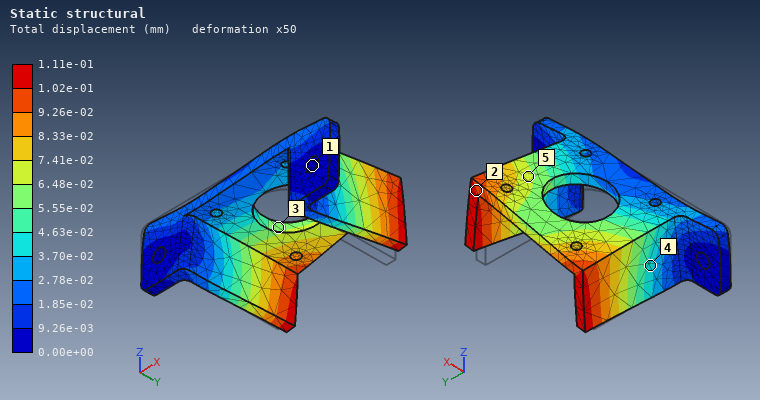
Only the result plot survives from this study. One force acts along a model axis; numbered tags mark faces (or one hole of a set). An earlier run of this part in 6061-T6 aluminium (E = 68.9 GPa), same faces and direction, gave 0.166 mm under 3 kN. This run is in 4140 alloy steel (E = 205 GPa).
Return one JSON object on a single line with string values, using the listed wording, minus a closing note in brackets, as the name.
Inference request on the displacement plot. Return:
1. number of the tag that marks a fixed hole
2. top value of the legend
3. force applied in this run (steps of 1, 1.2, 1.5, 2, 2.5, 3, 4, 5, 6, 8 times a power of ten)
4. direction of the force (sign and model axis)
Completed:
{"number of the tag that marks a fixed hole": "1", "top value of the legend": "1.11e-01 mm", "force applied in this run": "6 kN", "direction of the force": "+X"}
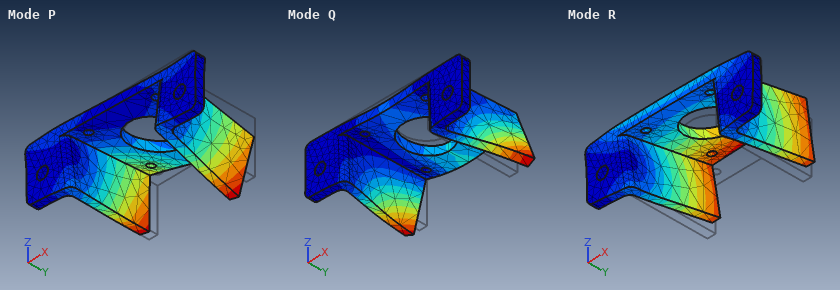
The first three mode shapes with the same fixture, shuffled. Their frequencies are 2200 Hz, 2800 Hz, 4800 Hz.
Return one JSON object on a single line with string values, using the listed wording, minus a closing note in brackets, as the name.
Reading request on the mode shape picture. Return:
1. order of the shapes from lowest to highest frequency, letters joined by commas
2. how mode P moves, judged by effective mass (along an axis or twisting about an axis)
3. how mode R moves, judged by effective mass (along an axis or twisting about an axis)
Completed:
{"order of the shapes from lowest to highest frequency, letters joined by commas": "R, P, Q", "how mode P moves, judged by effective mass": "along X", "how mode R moves, judged by effective mass": "along Z"}
